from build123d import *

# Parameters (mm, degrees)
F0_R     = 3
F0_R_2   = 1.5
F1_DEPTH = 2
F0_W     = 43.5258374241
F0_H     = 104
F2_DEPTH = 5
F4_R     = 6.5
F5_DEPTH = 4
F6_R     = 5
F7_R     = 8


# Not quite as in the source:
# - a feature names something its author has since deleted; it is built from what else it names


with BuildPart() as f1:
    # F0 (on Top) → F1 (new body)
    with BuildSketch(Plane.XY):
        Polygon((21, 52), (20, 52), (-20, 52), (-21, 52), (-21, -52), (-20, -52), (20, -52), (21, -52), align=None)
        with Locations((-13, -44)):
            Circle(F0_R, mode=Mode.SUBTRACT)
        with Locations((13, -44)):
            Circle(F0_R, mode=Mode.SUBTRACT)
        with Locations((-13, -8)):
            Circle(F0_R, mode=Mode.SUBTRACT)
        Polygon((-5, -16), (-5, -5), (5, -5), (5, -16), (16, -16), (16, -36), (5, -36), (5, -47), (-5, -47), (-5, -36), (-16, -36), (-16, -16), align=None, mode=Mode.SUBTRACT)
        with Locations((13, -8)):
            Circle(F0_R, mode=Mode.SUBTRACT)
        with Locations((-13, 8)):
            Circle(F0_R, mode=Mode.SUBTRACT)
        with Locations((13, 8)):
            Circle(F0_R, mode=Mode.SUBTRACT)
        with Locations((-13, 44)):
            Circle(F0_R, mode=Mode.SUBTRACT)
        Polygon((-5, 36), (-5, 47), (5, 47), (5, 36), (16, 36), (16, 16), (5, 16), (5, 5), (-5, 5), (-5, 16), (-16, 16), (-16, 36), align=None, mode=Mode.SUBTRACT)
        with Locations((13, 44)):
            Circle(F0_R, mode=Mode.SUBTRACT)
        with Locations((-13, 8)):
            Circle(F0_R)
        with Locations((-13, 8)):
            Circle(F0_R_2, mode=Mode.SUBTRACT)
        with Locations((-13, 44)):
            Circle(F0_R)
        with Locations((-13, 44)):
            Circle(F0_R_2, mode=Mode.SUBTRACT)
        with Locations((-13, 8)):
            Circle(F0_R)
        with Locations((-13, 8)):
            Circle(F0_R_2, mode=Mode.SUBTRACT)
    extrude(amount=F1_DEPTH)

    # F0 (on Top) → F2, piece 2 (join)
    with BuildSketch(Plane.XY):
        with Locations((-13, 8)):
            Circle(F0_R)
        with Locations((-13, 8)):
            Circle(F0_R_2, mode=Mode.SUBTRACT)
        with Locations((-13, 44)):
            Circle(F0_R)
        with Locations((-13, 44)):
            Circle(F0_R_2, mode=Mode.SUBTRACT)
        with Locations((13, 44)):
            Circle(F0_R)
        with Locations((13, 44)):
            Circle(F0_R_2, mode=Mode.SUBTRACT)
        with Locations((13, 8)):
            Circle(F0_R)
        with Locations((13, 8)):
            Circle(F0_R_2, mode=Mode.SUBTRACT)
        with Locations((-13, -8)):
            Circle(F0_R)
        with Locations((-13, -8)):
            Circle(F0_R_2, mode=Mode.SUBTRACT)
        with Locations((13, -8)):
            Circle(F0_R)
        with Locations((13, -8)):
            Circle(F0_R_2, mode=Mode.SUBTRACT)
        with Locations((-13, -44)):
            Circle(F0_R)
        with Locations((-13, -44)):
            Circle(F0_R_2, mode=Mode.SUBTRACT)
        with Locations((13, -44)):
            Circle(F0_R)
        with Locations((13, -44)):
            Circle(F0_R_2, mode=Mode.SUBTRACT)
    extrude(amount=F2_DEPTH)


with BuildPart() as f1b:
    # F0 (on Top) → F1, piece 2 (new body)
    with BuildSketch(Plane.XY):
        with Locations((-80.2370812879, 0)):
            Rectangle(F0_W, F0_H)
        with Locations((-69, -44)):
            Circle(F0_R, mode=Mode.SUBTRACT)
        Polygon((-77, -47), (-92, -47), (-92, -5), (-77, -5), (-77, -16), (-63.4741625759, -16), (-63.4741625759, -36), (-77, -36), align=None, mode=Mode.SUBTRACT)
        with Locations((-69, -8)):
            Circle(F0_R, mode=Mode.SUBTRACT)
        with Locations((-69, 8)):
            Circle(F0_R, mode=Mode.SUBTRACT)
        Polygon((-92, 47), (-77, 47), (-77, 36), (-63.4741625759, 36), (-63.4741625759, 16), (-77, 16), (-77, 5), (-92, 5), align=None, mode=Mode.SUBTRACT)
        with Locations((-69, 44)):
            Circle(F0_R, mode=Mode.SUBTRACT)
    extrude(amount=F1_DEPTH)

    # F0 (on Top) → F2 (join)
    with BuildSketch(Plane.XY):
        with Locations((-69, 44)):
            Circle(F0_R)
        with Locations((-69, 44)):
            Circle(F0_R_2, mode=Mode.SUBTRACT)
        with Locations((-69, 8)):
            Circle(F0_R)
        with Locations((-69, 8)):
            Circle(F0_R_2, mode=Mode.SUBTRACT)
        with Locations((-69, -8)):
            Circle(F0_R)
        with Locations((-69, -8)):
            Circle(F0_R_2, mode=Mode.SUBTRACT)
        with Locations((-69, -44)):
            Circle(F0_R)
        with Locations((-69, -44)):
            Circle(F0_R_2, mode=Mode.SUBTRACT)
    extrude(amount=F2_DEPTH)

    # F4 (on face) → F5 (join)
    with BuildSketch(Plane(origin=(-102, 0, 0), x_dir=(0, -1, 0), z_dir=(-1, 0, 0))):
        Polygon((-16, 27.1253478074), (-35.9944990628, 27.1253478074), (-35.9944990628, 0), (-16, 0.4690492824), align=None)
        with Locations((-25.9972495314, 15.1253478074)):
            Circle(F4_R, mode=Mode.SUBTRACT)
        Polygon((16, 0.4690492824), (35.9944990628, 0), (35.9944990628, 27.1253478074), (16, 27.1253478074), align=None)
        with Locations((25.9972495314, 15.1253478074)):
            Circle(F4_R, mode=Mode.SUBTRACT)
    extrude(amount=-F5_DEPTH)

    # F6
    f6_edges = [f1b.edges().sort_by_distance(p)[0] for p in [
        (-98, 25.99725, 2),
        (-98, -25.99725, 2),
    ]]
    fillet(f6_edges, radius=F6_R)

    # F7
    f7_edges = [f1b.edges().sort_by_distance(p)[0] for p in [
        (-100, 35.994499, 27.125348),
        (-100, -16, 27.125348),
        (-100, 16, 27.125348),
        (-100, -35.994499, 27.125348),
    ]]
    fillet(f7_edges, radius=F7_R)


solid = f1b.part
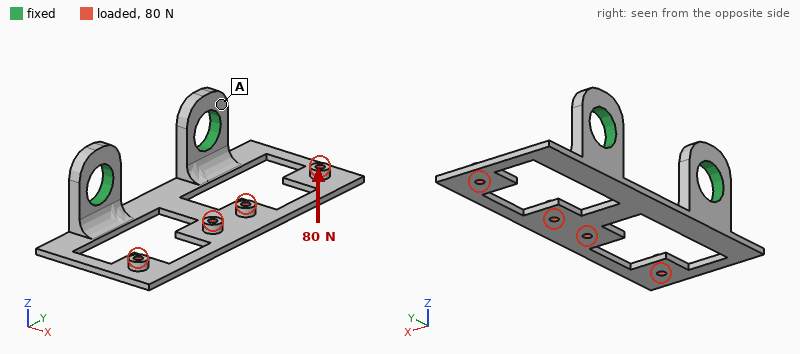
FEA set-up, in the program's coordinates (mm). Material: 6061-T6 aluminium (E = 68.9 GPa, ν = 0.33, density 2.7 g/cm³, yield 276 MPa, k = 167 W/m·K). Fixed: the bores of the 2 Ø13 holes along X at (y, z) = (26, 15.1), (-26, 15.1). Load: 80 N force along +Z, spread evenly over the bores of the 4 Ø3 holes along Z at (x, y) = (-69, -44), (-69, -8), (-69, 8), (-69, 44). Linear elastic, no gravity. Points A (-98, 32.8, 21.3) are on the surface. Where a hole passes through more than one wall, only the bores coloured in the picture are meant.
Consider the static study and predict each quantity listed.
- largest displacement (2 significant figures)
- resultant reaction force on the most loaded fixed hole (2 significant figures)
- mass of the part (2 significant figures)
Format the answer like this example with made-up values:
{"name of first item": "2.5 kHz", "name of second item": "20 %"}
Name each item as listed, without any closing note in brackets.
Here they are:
{"largest displacement": "1.3 mm", "resultant reaction force on the most loaded fixed hole": "41 N", "mass of the part": "23 g"}
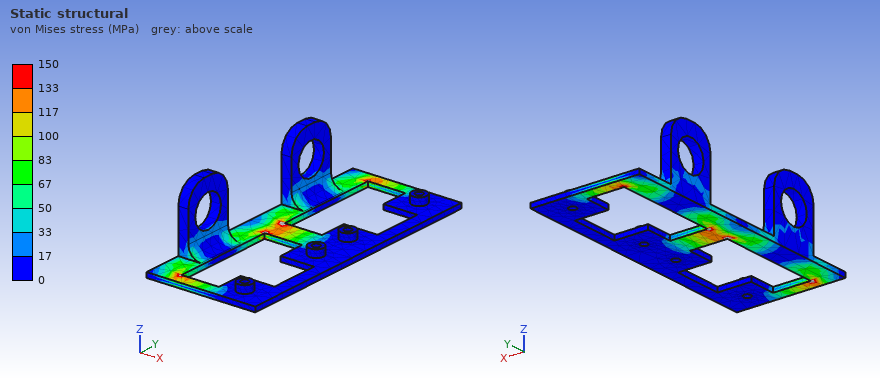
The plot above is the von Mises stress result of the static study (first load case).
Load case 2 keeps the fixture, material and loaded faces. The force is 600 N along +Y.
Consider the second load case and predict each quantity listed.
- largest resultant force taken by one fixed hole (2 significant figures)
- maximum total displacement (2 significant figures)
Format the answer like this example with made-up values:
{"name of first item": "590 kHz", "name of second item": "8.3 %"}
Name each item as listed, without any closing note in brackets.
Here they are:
{"largest resultant force taken by one fixed hole": "420 N", "maximum total displacement": "0.42 mm"}
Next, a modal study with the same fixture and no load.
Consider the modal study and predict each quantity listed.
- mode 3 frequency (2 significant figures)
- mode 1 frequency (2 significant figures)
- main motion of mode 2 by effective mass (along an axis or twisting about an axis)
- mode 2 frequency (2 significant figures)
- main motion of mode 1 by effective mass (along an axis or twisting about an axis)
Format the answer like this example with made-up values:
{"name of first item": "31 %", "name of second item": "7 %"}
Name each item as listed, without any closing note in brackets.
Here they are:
{"mode 3 frequency": "1300 Hz", "mode 1 frequency": "480 Hz", "main motion of mode 2 by effective mass": "twisting about X", "mode 2 frequency": "750 Hz", "main motion of mode 1 by effective mass": "along Z"}
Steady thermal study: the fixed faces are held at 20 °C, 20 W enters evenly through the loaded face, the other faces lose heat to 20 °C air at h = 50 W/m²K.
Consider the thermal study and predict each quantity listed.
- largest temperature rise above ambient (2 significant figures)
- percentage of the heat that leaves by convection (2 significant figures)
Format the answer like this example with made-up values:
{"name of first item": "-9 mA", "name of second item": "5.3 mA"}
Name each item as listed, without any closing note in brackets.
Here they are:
{"largest temperature rise above ambient": "53 K", "percentage of the heat that leaves by convection": "53 %"}
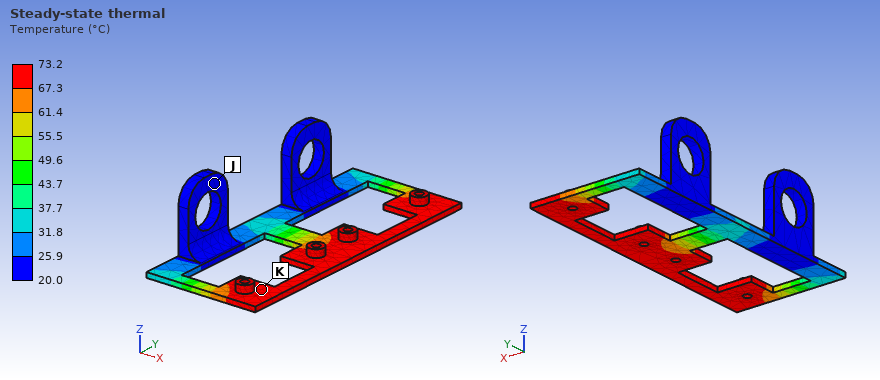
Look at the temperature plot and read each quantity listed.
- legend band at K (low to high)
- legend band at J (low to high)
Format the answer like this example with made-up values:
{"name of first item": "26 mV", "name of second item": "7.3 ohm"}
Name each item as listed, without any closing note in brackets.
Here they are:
{"legend band at K": "67.3 to 73.2 °C", "legend band at J": "20.0 to 25.9 °C"}
